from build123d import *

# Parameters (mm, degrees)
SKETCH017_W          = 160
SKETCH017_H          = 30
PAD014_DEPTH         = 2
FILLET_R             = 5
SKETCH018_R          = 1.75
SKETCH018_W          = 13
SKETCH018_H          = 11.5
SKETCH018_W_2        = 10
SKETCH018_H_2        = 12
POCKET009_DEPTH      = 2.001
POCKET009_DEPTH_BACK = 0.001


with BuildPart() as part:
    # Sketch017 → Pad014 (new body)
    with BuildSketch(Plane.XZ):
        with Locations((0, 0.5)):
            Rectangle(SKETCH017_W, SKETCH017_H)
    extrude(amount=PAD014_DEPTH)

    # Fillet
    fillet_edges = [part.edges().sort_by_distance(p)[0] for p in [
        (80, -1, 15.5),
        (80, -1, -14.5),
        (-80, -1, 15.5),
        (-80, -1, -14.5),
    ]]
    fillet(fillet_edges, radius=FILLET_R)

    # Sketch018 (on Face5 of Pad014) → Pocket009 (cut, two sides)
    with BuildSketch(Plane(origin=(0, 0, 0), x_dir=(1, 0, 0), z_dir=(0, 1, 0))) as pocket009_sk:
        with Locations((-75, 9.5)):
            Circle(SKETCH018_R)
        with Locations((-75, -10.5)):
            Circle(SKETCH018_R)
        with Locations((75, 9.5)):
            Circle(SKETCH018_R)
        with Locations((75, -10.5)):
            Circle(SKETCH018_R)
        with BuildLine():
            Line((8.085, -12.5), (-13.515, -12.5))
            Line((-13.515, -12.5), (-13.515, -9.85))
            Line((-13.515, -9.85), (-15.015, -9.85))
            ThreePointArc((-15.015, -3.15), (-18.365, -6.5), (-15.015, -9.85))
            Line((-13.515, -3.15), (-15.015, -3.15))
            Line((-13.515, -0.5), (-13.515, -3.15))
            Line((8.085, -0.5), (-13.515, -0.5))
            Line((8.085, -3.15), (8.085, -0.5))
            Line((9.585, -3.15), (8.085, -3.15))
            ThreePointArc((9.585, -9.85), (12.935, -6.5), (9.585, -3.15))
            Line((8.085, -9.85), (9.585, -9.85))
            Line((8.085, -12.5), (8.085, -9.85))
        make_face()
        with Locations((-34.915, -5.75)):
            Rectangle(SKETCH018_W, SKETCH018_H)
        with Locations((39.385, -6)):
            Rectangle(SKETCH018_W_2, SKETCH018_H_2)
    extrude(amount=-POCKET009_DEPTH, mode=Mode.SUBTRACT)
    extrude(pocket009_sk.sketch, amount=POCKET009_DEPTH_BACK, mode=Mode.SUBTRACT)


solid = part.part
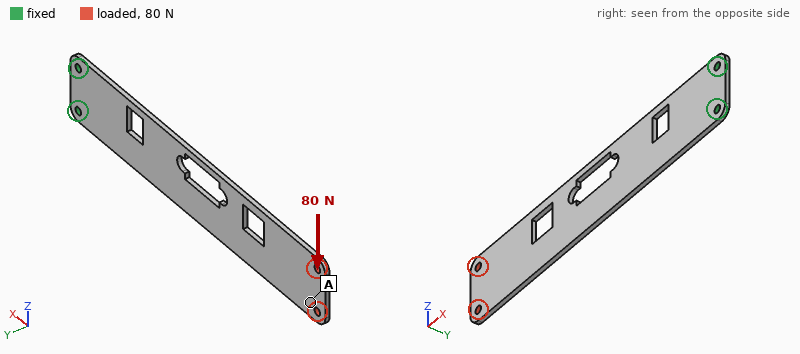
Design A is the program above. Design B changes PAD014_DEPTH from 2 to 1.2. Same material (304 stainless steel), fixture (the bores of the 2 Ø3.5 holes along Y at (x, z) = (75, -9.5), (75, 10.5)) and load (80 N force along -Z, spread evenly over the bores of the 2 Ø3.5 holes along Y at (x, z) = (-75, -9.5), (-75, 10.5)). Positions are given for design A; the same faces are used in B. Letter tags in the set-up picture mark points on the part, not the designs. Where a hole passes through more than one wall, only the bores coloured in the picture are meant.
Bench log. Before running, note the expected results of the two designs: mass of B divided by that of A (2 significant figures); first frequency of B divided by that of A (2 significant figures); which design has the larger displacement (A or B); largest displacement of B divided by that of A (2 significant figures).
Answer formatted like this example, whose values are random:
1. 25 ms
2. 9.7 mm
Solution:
1. 0.60
2. 0.60
3. B
4. 1.7
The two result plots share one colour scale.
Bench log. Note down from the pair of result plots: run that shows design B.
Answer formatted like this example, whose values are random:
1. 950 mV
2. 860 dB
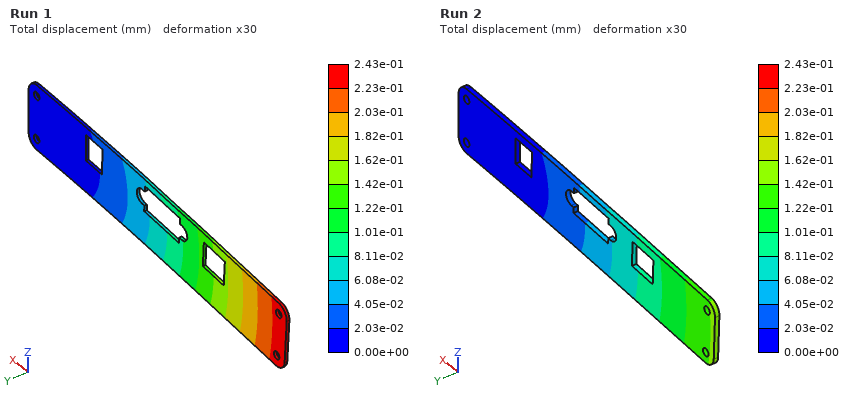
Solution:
1. Run 1
